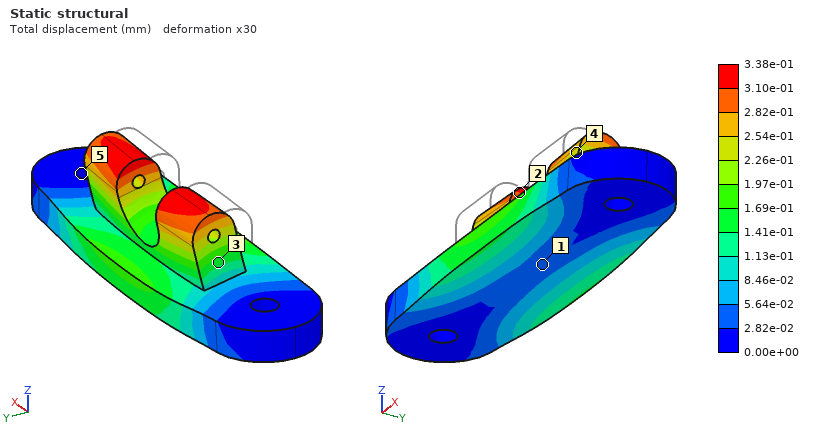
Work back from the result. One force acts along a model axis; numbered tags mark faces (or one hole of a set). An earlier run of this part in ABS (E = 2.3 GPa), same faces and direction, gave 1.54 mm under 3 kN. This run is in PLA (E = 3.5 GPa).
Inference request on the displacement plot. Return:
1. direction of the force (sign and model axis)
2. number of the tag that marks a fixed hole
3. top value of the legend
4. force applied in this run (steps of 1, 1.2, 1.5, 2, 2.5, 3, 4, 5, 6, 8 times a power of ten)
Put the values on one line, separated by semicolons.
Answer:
+Y; 5; 3.38e-01 mm; 1 kN
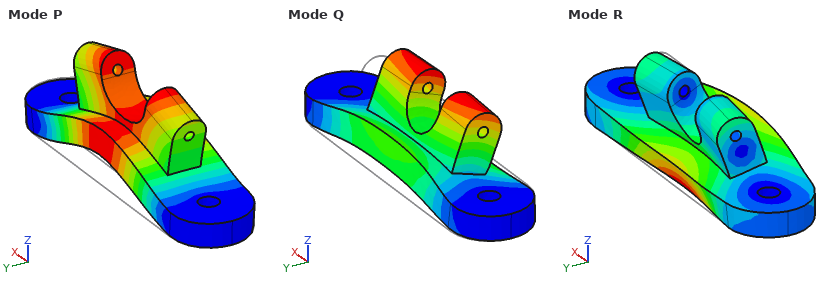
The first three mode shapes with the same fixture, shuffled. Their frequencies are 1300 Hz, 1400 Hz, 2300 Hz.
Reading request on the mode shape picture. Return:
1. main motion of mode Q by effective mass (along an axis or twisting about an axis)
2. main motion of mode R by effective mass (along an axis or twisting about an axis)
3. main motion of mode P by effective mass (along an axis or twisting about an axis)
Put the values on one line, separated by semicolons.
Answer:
along Y; along Y; along Z
